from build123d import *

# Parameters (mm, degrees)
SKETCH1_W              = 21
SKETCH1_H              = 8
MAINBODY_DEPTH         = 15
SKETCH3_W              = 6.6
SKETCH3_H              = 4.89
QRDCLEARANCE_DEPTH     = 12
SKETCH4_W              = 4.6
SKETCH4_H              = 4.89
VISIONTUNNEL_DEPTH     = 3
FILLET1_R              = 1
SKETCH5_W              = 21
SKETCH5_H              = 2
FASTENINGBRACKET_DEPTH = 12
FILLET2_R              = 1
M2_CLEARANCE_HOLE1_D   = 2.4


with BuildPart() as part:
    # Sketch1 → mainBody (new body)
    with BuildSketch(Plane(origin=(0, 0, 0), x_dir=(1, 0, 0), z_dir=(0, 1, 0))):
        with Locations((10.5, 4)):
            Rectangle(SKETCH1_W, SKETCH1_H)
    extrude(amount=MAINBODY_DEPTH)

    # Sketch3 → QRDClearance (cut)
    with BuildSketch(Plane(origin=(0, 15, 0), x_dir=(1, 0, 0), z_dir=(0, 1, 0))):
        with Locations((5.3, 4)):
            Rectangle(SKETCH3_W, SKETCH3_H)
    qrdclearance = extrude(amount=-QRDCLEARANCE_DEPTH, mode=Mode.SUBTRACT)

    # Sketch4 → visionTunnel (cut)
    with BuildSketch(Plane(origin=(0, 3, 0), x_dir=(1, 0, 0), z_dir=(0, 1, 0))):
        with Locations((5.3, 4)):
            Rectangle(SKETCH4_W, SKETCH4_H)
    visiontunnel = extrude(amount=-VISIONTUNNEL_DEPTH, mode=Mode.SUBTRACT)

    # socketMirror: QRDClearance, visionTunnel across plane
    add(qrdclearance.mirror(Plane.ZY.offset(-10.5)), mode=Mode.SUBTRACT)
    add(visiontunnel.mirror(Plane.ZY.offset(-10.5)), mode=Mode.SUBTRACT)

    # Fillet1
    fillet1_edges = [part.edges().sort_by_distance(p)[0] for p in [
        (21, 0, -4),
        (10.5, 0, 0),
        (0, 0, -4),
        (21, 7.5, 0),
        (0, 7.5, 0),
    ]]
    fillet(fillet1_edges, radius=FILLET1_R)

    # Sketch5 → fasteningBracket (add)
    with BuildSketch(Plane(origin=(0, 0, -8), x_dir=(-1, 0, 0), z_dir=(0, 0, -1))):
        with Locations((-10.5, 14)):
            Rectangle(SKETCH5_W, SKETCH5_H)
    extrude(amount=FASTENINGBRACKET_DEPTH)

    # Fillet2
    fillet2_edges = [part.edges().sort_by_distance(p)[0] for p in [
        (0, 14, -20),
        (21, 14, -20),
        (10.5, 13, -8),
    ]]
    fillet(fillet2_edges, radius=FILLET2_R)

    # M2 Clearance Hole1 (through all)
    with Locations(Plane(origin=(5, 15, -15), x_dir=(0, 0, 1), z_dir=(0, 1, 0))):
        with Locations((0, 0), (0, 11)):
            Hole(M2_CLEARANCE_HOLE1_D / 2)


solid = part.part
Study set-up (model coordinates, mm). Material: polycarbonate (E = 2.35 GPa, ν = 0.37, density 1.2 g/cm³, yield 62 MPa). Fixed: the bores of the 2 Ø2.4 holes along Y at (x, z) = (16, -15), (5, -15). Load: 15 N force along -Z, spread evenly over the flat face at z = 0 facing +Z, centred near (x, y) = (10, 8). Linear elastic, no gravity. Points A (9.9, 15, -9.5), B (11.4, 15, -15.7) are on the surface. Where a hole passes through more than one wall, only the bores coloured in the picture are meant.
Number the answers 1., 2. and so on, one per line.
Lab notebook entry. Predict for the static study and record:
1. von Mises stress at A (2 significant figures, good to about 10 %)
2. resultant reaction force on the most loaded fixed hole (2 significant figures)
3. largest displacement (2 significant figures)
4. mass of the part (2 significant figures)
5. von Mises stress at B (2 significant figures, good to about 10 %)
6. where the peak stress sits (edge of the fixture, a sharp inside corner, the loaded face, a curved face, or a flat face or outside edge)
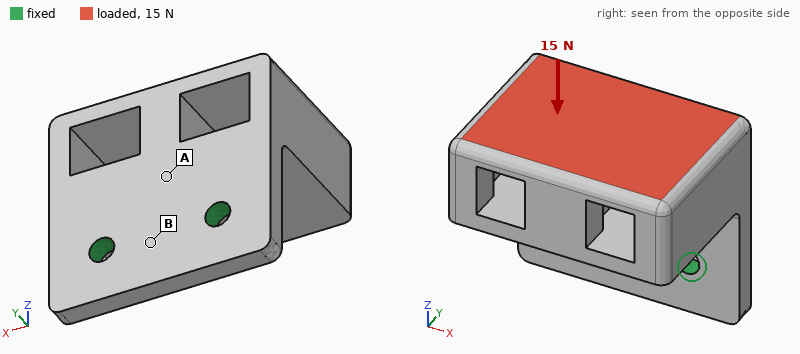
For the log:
1. 5.9 MPa
2. 7.6 N
3. 0.35 mm
4. 2.5 g
5. 1.6 MPa
6. a flat face or outside edge
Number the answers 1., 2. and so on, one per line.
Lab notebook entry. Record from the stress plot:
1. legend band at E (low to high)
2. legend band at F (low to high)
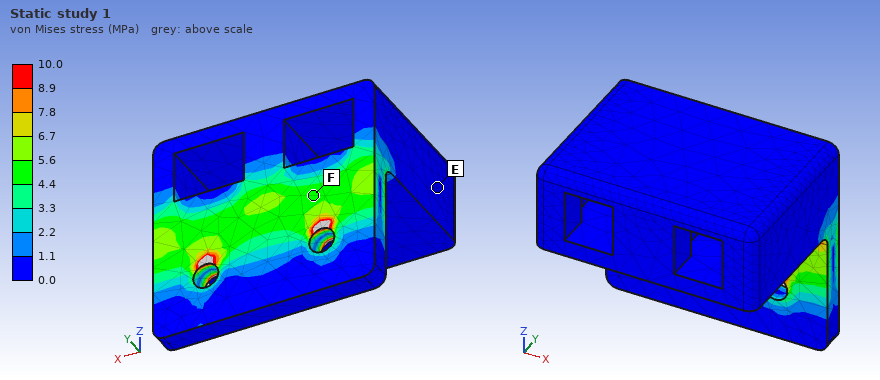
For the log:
1. 0.0 to 1.1 MPa
2. 4.4 to 5.6 MPa
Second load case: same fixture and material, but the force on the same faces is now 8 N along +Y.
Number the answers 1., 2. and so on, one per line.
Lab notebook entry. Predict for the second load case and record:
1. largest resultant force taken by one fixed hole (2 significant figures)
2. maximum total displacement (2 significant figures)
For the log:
1. 4.0 N
2. 0.35 mm
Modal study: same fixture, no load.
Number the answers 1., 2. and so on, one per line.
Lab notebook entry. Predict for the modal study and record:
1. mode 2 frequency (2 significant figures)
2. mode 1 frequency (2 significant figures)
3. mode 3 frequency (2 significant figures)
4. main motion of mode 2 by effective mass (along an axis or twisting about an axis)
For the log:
1. 1800 Hz
2. 700 Hz
3. 3700 Hz
4. along X
